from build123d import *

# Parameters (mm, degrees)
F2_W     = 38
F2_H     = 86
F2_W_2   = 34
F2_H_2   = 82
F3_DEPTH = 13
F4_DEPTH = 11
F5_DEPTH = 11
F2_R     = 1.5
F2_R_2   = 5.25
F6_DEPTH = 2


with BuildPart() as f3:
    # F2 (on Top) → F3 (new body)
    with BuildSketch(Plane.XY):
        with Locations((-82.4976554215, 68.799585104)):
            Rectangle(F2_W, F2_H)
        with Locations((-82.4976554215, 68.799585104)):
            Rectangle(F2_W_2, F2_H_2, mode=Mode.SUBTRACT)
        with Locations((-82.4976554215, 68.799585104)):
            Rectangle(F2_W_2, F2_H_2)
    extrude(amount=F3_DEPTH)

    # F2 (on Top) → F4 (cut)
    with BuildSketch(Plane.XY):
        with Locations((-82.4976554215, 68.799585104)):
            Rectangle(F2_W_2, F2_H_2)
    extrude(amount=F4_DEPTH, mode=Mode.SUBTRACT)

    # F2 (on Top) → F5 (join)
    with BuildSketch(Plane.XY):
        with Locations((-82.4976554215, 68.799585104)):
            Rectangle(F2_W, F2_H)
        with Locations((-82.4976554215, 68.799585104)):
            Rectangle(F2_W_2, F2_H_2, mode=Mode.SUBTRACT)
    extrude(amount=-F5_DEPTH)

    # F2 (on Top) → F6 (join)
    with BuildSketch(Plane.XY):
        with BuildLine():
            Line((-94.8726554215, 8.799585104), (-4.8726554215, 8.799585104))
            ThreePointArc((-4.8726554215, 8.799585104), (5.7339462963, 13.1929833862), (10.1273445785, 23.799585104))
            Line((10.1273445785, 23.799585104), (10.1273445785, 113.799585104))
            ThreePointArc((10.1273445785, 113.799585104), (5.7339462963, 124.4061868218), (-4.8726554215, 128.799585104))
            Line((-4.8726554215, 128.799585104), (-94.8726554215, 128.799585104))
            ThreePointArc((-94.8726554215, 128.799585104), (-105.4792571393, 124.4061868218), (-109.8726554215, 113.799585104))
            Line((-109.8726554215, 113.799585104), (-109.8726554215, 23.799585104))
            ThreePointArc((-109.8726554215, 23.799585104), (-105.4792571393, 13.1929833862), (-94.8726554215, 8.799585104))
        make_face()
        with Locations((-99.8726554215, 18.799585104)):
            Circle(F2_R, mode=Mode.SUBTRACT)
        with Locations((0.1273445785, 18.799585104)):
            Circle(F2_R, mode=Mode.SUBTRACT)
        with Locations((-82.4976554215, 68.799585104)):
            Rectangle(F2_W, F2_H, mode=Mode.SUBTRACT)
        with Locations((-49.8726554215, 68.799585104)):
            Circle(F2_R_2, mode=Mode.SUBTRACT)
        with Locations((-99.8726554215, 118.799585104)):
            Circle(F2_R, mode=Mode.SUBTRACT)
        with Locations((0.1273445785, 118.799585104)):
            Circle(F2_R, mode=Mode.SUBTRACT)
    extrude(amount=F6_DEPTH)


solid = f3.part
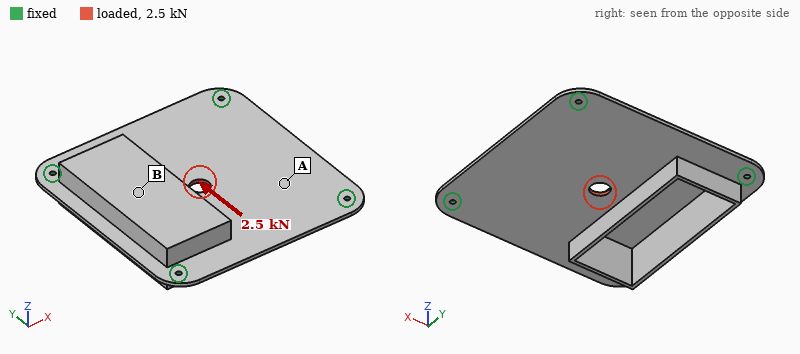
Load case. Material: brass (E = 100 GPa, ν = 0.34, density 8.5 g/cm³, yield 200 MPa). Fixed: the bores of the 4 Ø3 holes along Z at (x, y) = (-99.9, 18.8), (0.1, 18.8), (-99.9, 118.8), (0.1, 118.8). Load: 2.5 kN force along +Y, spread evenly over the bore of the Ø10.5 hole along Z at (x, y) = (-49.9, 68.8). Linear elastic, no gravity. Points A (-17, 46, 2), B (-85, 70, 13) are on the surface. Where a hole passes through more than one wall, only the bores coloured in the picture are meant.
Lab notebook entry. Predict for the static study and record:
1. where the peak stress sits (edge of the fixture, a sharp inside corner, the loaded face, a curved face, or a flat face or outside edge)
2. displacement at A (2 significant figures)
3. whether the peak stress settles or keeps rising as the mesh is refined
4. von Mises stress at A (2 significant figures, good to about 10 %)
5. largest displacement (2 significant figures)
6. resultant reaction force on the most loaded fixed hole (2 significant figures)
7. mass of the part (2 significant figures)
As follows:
edge of the fixture
12 µm
keeps rising
15 MPa
56 µm
1.2 kN
330 g
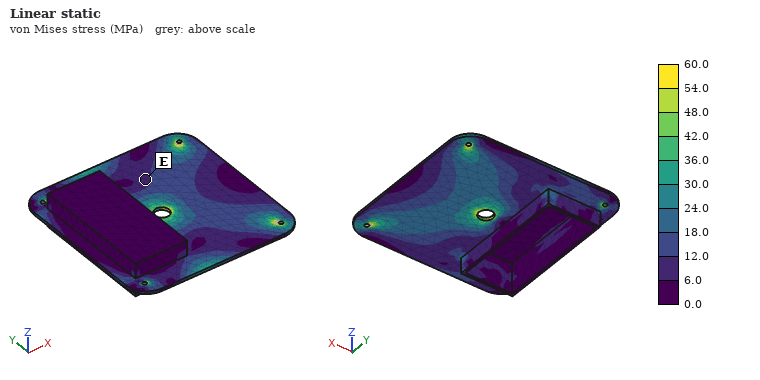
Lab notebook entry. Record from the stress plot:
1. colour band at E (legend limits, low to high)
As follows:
6.0 to 12.0 MPa
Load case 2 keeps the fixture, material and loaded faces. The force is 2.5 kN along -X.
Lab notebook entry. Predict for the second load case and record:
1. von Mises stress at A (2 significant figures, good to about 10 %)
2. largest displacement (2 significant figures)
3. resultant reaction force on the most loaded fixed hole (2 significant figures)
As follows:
16 MPa
33 µm
900 N
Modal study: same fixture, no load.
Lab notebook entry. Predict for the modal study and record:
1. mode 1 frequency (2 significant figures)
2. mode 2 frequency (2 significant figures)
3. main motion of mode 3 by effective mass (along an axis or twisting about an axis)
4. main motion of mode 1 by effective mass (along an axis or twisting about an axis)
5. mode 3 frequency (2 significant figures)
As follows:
480 Hz
810 Hz
twisting about X
along Z
1300 Hz
